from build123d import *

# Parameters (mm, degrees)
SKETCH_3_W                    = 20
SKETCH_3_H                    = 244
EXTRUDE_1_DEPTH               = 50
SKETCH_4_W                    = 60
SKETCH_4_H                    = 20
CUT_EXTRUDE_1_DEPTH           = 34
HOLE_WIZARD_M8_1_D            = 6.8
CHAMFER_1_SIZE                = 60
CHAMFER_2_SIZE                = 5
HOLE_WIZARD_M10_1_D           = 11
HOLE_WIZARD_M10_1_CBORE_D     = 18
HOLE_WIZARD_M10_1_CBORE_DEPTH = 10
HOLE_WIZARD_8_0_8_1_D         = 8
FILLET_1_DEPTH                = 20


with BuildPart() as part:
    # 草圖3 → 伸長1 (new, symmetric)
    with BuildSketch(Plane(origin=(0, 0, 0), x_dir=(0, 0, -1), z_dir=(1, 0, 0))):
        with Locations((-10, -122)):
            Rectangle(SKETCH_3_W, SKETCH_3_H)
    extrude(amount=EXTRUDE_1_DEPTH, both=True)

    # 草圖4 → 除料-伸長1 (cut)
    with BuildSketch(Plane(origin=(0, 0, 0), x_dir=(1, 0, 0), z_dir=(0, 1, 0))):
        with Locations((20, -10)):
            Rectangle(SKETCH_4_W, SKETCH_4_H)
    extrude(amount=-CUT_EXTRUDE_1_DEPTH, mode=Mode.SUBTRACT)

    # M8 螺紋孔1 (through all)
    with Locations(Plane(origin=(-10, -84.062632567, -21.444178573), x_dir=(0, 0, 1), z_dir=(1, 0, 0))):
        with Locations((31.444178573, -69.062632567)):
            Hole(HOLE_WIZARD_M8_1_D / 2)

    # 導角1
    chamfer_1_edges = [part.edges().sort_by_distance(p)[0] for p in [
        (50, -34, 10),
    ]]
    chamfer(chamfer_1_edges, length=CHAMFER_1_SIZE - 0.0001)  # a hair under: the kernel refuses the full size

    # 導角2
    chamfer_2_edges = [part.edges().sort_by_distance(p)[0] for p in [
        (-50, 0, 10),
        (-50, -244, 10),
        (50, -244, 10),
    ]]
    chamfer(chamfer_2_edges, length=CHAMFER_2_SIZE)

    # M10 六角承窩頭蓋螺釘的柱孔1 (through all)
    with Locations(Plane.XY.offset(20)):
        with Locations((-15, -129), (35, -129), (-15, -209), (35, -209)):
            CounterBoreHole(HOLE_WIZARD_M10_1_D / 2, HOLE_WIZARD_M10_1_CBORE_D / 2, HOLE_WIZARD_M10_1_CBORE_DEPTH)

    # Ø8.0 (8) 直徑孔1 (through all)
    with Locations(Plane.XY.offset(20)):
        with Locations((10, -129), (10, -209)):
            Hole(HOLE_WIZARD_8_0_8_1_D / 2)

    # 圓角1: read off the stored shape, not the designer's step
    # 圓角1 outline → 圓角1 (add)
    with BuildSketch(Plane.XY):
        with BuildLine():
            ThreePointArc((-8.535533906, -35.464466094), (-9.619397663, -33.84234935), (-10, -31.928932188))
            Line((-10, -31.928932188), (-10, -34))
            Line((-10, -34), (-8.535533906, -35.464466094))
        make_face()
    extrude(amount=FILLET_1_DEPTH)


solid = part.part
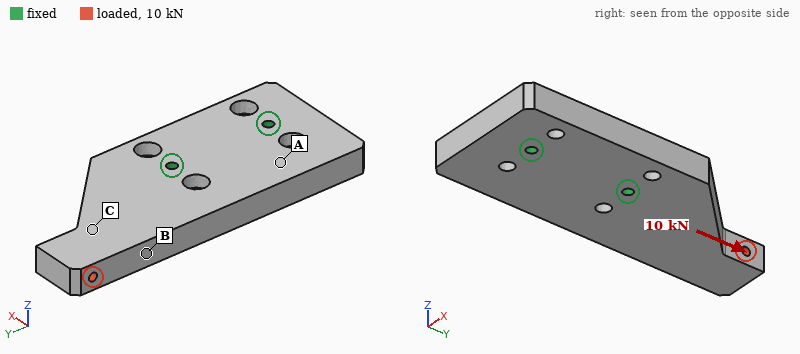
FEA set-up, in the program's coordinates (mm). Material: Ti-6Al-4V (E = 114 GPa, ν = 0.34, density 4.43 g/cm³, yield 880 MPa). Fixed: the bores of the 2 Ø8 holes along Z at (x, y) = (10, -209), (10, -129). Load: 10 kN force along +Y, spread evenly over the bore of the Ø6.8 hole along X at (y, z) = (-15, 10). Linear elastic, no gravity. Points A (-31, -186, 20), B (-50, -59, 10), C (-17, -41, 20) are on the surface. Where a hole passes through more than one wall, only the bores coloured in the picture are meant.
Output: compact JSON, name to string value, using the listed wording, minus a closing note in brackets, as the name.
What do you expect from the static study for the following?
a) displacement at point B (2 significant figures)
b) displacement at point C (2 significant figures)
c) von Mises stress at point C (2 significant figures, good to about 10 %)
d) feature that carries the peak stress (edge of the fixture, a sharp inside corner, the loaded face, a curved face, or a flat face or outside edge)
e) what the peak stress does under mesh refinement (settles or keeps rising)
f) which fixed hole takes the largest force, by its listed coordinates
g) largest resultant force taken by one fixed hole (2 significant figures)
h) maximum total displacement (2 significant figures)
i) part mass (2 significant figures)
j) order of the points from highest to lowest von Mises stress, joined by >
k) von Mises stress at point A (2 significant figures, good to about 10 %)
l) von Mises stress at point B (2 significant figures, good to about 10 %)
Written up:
{"displacement at point B": "26 µm", "displacement at point C": "24 µm", "von Mises stress at point C": "11 MPa", "feature that carries the peak stress": "edge of the fixture", "what the peak stress does under mesh refinement": "keeps rising", "which fixed hole takes the largest force, by its listed coordinates": "(10, -129)", "largest resultant force taken by one fixed hole": "8.0 kN", "maximum total displacement": "43 µm", "part mass": "1.7 kg", "order of the points from highest to lowest von Mises stress, joined by >": "B > C > A", "von Mises stress at point A": "4.7 MPa", "von Mises stress at point B": "16 MPa"}
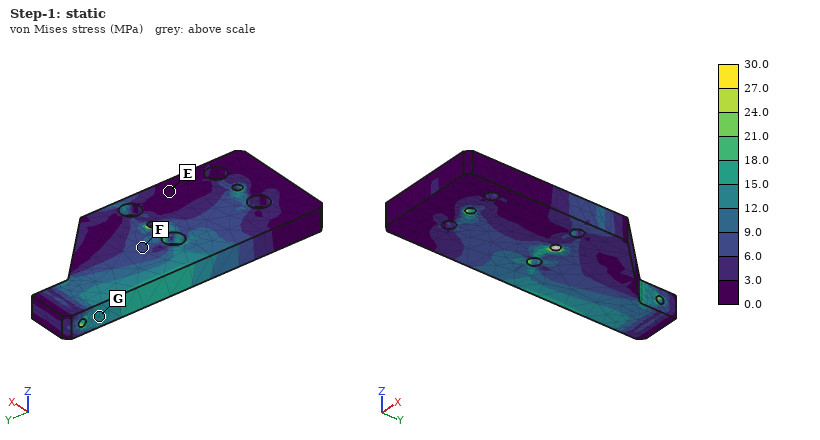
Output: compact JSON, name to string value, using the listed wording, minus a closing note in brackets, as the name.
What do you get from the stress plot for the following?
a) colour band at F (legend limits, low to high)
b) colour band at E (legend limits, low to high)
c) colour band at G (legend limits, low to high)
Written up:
{"colour band at F": "6.0 to 9.0 MPa", "colour band at E": "0.0 to 3.0 MPa", "colour band at G": "12.0 to 15.0 MPa"}
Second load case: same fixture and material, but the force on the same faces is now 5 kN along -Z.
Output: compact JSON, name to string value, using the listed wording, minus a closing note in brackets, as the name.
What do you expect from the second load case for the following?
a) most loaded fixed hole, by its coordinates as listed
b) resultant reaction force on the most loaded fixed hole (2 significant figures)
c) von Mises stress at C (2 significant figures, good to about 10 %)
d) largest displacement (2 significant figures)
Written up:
{"most loaded fixed hole, by its coordinates as listed": "(10, -129)", "resultant reaction force on the most loaded fixed hole": "8.4 kN", "von Mises stress at C": "56 MPa", "largest displacement": "0.75 mm"}
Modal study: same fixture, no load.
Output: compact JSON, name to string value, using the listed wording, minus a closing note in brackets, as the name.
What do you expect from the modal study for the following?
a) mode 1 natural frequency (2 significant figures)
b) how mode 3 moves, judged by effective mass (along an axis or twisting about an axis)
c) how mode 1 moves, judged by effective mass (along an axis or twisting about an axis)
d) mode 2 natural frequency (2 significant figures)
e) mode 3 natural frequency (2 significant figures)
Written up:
{"mode 1 natural frequency": "1100 Hz", "how mode 3 moves, judged by effective mass": "along X", "how mode 1 moves, judged by effective mass": "along Z", "mode 2 natural frequency": "2800 Hz", "mode 3 natural frequency": "2900 Hz"}
